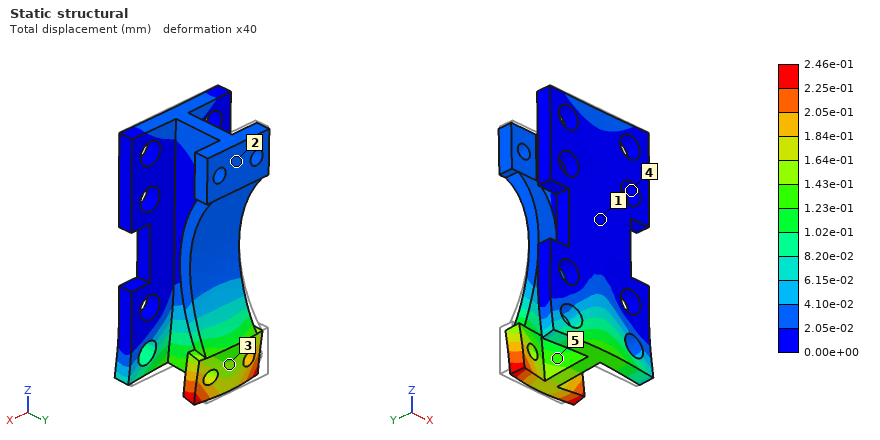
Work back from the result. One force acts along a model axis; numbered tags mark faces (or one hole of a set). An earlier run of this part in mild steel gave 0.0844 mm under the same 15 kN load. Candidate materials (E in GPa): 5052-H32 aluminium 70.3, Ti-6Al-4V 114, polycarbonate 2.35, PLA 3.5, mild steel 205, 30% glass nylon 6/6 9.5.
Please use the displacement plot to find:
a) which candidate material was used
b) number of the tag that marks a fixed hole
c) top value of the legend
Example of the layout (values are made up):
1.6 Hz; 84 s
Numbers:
5052-H32 aluminium; 4; 2.46e-01 mm
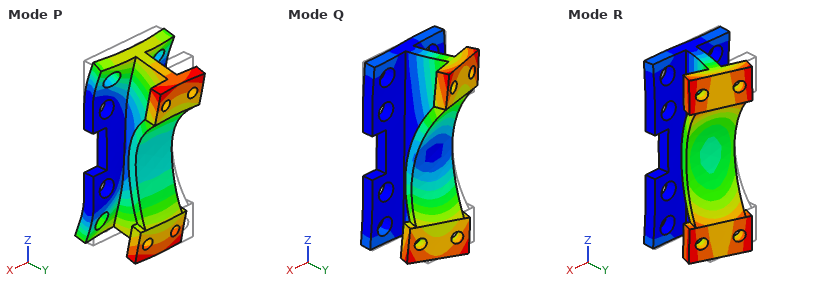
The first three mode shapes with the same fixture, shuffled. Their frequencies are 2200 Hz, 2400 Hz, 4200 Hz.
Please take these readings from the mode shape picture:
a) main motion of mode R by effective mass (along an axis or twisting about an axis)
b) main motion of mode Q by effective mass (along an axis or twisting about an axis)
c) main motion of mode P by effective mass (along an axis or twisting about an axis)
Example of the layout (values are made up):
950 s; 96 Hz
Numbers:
along X; twisting about Y; along Z
